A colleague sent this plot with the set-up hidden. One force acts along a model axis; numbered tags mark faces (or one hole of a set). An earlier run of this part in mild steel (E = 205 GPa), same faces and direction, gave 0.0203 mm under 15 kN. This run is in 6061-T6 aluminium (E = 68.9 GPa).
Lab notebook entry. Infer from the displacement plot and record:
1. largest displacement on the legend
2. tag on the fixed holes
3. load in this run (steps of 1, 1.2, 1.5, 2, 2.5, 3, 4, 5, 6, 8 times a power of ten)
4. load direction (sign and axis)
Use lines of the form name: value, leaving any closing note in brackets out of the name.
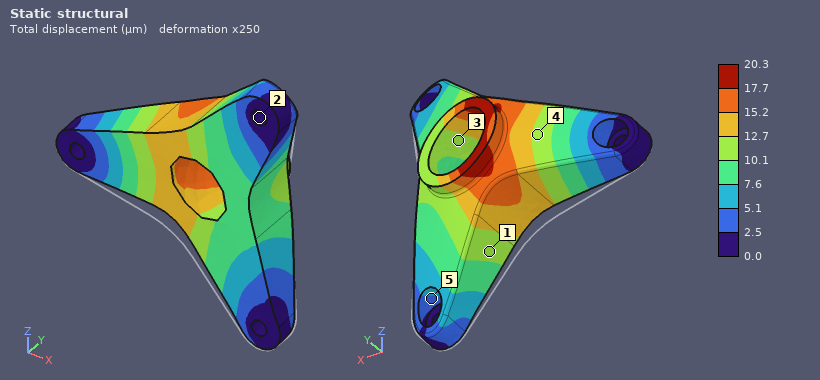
largest displacement on the legend: 20.3 µm
tag on the fixed holes: 2
load in this run: 5 kN
load direction: +Z
